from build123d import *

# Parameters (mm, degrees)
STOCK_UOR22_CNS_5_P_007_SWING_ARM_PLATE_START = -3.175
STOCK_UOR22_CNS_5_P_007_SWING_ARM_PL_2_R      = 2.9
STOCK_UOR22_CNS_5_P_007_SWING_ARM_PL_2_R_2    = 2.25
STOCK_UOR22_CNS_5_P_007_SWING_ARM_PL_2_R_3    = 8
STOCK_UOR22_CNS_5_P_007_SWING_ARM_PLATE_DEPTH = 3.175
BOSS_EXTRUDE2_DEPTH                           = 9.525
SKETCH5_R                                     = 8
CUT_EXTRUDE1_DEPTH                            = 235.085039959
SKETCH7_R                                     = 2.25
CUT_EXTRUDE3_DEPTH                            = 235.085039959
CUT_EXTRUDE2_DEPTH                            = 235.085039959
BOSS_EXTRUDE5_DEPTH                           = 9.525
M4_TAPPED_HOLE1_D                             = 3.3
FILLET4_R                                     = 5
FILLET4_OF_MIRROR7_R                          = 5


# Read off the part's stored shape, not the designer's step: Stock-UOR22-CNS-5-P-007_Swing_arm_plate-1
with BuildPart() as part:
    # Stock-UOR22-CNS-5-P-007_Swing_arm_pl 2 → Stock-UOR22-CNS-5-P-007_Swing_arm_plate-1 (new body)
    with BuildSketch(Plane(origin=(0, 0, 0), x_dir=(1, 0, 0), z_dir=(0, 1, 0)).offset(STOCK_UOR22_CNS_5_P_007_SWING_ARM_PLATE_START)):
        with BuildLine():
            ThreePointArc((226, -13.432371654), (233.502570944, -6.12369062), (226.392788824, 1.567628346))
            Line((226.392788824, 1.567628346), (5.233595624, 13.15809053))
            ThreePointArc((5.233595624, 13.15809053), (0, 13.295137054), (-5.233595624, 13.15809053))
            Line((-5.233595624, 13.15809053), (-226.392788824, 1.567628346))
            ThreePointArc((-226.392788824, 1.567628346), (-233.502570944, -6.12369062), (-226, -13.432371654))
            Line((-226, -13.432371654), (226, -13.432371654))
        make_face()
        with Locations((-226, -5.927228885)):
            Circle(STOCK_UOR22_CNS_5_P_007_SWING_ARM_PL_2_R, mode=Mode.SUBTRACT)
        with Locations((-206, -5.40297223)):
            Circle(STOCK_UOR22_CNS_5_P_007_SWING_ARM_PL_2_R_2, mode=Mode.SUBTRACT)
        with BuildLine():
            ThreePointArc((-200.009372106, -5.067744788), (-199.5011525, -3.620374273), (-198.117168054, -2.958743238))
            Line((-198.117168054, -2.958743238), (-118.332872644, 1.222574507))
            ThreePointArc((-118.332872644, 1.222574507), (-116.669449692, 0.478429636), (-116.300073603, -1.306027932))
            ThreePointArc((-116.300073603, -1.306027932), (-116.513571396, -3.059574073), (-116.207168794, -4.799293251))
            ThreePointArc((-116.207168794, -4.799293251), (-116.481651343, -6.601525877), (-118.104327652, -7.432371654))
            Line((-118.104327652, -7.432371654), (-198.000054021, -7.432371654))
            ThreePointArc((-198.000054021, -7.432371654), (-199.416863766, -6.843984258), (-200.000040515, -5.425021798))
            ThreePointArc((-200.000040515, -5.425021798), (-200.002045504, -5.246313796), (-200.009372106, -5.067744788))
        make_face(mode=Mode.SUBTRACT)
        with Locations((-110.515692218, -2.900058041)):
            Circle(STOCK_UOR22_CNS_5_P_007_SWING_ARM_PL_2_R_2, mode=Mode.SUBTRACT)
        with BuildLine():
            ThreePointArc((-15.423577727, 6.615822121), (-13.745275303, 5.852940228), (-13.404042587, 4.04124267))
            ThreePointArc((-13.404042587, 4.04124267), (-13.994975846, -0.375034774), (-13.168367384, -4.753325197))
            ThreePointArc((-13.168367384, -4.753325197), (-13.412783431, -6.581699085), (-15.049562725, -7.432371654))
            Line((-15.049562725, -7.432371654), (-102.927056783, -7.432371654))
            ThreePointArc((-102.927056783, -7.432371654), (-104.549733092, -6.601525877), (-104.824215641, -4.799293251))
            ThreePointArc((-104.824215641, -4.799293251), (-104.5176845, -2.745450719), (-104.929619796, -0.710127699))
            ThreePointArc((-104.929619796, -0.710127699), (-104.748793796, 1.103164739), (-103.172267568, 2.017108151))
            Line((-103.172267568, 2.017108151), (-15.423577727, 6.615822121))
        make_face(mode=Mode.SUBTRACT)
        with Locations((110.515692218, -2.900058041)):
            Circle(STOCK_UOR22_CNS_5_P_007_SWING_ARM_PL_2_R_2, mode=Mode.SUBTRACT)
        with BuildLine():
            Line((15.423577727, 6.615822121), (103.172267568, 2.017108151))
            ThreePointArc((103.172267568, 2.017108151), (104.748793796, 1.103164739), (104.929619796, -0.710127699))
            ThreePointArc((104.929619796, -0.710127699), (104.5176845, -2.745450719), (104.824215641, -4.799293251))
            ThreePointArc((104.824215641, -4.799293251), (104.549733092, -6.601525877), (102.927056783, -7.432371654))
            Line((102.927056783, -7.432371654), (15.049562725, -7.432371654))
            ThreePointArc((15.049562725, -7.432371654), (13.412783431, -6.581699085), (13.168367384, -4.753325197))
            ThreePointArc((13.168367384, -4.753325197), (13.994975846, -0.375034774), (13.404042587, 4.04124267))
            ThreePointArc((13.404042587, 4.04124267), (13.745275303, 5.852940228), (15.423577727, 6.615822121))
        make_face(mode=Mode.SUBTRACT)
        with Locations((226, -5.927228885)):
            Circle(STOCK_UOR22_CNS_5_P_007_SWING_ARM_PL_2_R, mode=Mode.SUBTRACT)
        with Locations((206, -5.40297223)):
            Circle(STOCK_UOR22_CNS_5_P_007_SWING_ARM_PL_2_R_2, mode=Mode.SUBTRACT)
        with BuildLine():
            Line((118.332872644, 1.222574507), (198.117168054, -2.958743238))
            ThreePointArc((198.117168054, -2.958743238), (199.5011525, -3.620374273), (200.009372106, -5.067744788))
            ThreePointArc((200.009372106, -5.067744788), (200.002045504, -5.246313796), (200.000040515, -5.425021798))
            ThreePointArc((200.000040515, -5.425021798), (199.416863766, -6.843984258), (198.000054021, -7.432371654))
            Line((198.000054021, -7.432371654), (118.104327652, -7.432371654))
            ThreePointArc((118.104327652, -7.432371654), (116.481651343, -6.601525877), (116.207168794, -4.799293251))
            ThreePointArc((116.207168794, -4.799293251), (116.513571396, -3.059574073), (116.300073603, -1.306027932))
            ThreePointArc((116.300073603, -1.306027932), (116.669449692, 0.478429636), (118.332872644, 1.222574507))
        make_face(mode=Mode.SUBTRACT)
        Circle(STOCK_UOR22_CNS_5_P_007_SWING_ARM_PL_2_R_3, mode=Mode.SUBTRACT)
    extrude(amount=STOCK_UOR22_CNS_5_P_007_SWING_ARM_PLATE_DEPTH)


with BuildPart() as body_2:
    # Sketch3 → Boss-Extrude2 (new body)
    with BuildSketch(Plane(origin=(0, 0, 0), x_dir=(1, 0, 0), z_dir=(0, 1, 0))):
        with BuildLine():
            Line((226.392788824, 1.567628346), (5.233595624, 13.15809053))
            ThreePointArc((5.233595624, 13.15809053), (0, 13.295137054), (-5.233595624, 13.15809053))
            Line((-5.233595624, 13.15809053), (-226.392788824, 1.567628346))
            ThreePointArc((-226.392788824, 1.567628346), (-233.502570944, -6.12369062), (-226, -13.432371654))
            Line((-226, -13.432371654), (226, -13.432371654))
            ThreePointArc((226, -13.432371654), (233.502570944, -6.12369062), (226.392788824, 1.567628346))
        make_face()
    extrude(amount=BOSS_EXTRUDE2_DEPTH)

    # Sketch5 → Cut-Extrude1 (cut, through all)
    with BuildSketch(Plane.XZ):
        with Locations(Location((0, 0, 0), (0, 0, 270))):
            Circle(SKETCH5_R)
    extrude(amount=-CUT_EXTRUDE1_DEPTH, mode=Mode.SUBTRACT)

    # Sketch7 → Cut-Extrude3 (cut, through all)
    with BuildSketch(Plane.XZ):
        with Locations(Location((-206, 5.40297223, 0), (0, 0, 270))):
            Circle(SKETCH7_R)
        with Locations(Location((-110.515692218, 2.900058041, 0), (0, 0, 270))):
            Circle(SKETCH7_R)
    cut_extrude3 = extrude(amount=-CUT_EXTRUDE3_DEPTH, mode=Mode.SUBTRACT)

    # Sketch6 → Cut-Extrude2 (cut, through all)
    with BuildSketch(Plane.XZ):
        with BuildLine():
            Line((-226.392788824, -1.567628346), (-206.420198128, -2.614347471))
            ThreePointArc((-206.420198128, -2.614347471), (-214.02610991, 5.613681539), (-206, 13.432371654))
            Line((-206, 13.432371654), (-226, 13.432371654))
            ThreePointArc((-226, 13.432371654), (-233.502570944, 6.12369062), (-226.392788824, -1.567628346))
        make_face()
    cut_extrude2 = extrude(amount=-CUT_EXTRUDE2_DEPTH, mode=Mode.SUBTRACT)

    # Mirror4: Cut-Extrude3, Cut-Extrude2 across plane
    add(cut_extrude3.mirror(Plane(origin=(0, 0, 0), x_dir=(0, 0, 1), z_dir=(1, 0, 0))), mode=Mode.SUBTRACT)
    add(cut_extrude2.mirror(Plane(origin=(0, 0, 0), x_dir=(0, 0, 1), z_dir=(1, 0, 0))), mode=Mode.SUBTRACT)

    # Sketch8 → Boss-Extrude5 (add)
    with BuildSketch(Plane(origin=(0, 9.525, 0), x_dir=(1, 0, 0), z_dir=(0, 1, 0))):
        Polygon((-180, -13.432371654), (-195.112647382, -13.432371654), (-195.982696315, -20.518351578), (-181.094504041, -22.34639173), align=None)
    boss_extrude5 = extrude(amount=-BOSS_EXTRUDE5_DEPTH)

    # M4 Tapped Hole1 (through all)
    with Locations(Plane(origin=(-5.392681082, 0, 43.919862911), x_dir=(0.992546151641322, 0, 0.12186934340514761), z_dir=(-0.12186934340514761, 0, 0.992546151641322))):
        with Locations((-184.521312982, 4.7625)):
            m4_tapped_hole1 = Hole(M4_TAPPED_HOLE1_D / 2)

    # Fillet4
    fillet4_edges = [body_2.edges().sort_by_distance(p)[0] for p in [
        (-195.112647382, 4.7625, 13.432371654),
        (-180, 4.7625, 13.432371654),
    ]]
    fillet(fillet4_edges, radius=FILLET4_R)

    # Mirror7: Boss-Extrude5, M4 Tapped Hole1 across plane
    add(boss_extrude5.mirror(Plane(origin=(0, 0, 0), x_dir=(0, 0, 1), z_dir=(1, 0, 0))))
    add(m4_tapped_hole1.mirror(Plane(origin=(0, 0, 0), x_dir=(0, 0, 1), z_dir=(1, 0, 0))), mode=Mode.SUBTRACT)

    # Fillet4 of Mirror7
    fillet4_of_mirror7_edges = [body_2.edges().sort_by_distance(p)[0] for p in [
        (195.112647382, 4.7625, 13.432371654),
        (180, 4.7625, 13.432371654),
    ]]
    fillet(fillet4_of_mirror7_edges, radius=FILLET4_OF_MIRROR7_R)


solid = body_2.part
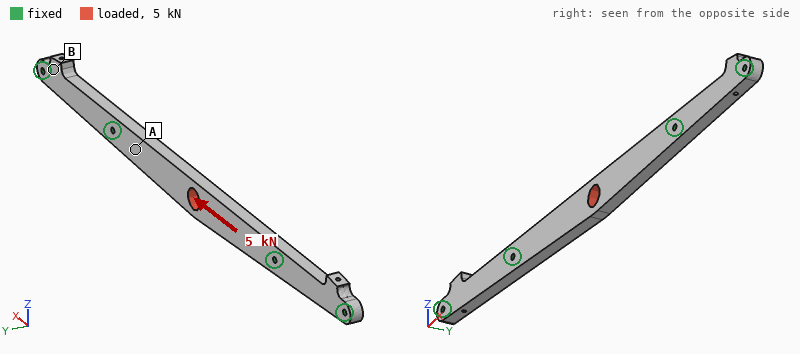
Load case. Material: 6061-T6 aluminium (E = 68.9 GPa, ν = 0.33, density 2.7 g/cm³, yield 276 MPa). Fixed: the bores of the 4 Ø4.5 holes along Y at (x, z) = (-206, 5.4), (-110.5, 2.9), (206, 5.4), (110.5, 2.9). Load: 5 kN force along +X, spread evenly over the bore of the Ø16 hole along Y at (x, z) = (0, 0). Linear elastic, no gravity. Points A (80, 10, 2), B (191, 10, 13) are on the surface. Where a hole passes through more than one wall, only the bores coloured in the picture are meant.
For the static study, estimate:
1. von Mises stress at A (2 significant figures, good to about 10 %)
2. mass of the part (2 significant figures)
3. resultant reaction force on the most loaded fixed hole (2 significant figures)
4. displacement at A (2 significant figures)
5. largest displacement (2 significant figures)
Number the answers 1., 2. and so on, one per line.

1. 12 MPa
2. 230 g
3. 2.4 kN
4. 6.0 µm
5. 19 µm
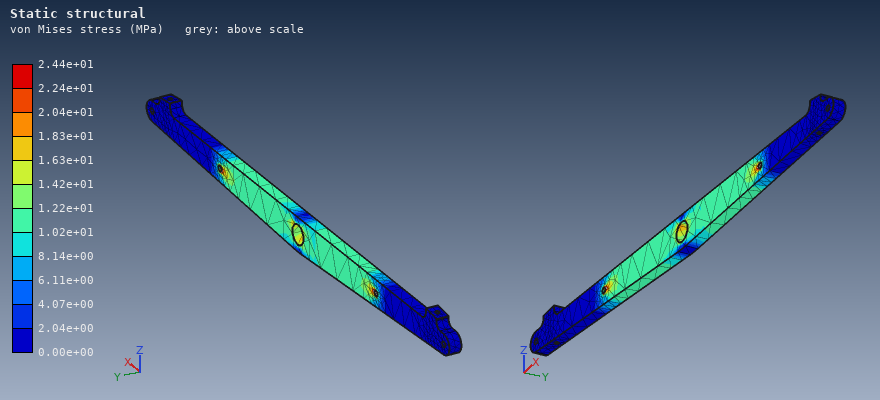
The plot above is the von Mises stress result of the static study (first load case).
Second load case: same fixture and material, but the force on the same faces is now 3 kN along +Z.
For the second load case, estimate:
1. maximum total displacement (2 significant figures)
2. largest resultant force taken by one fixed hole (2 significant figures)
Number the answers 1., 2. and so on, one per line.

1. 0.35 mm
2. 2.1 kN
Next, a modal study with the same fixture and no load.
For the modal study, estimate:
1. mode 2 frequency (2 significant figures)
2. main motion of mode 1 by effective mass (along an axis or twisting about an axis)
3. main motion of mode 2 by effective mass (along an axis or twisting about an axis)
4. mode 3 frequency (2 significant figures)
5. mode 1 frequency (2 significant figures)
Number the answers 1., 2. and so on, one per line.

1. 1900 Hz
2. along Y
3. along Z
4. 2600 Hz
5. 930 Hz
